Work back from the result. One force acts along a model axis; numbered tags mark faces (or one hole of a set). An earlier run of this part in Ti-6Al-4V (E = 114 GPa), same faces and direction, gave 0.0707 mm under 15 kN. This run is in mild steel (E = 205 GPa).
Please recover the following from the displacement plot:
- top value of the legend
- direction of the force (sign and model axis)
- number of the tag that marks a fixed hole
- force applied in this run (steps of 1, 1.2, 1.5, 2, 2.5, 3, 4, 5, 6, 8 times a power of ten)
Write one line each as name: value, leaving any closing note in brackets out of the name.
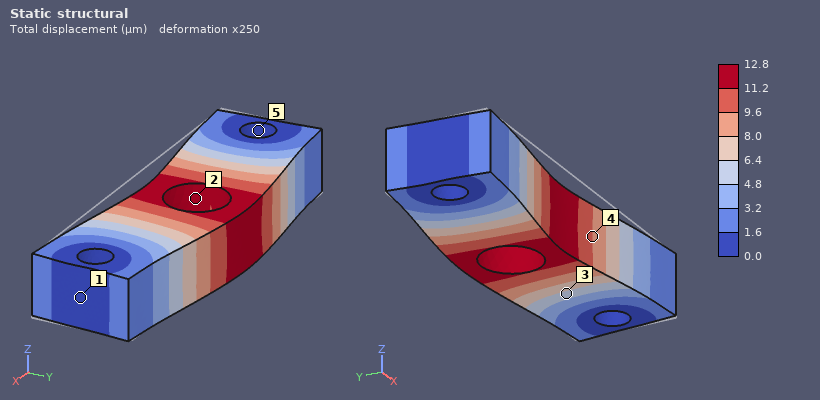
top value of the legend: 12.8 µm
direction of the force: +Y
number of the tag that marks a fixed hole: 5
force applied in this run: 5 kN
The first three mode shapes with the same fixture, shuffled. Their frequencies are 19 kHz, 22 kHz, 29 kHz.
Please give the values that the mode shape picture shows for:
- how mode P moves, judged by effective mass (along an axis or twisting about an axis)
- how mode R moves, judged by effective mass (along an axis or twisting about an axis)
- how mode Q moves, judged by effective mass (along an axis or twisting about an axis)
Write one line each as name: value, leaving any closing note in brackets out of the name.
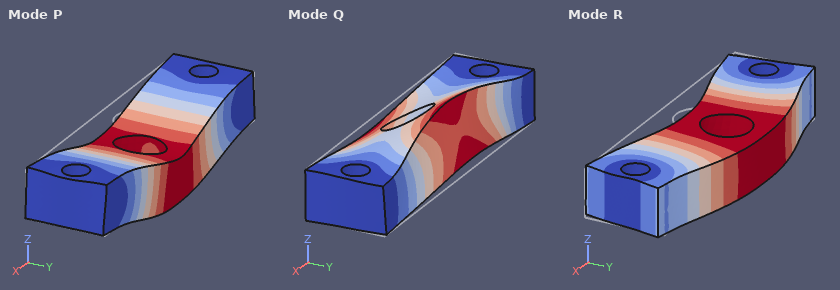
how mode P moves, judged by effective mass: along Z
how mode R moves, judged by effective mass: along Y
how mode Q moves, judged by effective mass: twisting about X
